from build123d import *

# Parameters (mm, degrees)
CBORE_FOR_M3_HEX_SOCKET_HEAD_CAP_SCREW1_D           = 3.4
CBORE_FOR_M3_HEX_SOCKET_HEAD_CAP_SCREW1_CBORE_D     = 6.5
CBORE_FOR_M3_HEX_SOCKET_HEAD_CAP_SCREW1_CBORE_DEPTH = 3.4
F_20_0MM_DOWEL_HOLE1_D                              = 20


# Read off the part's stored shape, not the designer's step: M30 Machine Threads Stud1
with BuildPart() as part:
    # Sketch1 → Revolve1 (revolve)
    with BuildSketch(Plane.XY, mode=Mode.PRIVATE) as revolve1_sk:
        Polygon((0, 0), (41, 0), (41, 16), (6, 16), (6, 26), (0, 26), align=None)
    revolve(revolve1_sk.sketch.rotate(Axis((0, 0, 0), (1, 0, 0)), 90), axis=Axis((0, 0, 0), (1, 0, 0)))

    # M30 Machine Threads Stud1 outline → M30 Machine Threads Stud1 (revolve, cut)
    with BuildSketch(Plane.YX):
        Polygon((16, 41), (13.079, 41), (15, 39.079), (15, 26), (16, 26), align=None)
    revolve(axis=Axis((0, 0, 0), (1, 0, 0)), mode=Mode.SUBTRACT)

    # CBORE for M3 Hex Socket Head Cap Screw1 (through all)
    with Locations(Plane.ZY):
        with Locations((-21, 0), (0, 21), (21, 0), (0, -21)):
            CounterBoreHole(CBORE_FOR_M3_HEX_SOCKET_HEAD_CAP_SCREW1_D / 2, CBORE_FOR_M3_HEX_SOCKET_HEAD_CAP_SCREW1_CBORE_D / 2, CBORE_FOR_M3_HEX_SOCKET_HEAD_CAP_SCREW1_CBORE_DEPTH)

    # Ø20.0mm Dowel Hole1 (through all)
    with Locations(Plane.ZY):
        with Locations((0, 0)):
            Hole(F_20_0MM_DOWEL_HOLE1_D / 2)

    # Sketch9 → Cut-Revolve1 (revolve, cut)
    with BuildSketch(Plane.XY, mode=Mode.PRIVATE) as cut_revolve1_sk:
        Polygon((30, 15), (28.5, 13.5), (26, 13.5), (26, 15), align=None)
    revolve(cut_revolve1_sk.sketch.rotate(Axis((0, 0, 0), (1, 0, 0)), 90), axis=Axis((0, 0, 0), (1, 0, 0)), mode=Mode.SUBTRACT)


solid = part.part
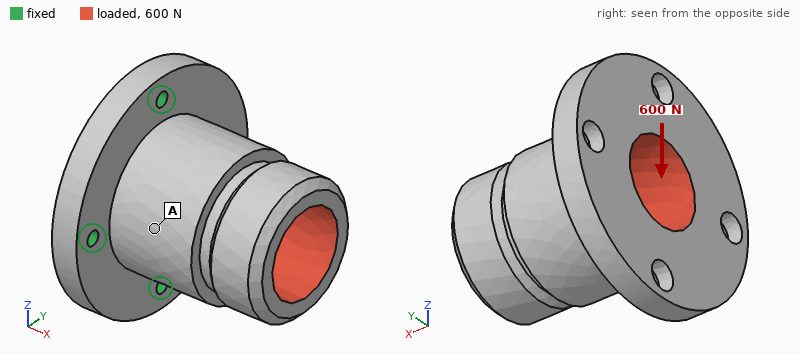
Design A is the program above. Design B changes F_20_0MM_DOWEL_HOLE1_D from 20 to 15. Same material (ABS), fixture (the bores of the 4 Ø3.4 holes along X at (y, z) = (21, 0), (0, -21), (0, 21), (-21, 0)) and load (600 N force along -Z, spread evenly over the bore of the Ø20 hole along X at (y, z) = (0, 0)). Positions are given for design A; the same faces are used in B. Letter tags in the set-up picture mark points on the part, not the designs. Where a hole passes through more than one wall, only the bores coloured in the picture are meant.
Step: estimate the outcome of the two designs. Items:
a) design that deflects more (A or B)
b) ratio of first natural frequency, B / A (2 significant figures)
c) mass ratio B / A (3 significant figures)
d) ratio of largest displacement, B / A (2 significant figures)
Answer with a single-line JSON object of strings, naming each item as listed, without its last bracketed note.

{"design that deflects more": "A", "ratio of first natural frequency, B / A": "0.91", "mass ratio B / A": "1.22", "ratio of largest displacement, B / A": "0.90"}
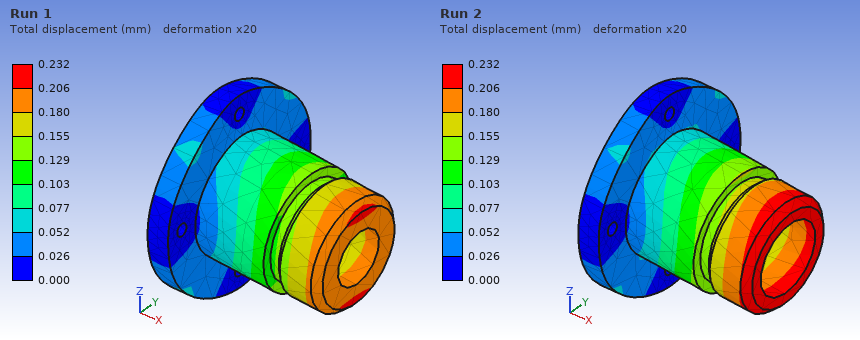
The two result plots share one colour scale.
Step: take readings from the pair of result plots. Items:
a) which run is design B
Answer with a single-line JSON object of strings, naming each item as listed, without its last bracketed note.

{"which run is design B": "Run 1"}
